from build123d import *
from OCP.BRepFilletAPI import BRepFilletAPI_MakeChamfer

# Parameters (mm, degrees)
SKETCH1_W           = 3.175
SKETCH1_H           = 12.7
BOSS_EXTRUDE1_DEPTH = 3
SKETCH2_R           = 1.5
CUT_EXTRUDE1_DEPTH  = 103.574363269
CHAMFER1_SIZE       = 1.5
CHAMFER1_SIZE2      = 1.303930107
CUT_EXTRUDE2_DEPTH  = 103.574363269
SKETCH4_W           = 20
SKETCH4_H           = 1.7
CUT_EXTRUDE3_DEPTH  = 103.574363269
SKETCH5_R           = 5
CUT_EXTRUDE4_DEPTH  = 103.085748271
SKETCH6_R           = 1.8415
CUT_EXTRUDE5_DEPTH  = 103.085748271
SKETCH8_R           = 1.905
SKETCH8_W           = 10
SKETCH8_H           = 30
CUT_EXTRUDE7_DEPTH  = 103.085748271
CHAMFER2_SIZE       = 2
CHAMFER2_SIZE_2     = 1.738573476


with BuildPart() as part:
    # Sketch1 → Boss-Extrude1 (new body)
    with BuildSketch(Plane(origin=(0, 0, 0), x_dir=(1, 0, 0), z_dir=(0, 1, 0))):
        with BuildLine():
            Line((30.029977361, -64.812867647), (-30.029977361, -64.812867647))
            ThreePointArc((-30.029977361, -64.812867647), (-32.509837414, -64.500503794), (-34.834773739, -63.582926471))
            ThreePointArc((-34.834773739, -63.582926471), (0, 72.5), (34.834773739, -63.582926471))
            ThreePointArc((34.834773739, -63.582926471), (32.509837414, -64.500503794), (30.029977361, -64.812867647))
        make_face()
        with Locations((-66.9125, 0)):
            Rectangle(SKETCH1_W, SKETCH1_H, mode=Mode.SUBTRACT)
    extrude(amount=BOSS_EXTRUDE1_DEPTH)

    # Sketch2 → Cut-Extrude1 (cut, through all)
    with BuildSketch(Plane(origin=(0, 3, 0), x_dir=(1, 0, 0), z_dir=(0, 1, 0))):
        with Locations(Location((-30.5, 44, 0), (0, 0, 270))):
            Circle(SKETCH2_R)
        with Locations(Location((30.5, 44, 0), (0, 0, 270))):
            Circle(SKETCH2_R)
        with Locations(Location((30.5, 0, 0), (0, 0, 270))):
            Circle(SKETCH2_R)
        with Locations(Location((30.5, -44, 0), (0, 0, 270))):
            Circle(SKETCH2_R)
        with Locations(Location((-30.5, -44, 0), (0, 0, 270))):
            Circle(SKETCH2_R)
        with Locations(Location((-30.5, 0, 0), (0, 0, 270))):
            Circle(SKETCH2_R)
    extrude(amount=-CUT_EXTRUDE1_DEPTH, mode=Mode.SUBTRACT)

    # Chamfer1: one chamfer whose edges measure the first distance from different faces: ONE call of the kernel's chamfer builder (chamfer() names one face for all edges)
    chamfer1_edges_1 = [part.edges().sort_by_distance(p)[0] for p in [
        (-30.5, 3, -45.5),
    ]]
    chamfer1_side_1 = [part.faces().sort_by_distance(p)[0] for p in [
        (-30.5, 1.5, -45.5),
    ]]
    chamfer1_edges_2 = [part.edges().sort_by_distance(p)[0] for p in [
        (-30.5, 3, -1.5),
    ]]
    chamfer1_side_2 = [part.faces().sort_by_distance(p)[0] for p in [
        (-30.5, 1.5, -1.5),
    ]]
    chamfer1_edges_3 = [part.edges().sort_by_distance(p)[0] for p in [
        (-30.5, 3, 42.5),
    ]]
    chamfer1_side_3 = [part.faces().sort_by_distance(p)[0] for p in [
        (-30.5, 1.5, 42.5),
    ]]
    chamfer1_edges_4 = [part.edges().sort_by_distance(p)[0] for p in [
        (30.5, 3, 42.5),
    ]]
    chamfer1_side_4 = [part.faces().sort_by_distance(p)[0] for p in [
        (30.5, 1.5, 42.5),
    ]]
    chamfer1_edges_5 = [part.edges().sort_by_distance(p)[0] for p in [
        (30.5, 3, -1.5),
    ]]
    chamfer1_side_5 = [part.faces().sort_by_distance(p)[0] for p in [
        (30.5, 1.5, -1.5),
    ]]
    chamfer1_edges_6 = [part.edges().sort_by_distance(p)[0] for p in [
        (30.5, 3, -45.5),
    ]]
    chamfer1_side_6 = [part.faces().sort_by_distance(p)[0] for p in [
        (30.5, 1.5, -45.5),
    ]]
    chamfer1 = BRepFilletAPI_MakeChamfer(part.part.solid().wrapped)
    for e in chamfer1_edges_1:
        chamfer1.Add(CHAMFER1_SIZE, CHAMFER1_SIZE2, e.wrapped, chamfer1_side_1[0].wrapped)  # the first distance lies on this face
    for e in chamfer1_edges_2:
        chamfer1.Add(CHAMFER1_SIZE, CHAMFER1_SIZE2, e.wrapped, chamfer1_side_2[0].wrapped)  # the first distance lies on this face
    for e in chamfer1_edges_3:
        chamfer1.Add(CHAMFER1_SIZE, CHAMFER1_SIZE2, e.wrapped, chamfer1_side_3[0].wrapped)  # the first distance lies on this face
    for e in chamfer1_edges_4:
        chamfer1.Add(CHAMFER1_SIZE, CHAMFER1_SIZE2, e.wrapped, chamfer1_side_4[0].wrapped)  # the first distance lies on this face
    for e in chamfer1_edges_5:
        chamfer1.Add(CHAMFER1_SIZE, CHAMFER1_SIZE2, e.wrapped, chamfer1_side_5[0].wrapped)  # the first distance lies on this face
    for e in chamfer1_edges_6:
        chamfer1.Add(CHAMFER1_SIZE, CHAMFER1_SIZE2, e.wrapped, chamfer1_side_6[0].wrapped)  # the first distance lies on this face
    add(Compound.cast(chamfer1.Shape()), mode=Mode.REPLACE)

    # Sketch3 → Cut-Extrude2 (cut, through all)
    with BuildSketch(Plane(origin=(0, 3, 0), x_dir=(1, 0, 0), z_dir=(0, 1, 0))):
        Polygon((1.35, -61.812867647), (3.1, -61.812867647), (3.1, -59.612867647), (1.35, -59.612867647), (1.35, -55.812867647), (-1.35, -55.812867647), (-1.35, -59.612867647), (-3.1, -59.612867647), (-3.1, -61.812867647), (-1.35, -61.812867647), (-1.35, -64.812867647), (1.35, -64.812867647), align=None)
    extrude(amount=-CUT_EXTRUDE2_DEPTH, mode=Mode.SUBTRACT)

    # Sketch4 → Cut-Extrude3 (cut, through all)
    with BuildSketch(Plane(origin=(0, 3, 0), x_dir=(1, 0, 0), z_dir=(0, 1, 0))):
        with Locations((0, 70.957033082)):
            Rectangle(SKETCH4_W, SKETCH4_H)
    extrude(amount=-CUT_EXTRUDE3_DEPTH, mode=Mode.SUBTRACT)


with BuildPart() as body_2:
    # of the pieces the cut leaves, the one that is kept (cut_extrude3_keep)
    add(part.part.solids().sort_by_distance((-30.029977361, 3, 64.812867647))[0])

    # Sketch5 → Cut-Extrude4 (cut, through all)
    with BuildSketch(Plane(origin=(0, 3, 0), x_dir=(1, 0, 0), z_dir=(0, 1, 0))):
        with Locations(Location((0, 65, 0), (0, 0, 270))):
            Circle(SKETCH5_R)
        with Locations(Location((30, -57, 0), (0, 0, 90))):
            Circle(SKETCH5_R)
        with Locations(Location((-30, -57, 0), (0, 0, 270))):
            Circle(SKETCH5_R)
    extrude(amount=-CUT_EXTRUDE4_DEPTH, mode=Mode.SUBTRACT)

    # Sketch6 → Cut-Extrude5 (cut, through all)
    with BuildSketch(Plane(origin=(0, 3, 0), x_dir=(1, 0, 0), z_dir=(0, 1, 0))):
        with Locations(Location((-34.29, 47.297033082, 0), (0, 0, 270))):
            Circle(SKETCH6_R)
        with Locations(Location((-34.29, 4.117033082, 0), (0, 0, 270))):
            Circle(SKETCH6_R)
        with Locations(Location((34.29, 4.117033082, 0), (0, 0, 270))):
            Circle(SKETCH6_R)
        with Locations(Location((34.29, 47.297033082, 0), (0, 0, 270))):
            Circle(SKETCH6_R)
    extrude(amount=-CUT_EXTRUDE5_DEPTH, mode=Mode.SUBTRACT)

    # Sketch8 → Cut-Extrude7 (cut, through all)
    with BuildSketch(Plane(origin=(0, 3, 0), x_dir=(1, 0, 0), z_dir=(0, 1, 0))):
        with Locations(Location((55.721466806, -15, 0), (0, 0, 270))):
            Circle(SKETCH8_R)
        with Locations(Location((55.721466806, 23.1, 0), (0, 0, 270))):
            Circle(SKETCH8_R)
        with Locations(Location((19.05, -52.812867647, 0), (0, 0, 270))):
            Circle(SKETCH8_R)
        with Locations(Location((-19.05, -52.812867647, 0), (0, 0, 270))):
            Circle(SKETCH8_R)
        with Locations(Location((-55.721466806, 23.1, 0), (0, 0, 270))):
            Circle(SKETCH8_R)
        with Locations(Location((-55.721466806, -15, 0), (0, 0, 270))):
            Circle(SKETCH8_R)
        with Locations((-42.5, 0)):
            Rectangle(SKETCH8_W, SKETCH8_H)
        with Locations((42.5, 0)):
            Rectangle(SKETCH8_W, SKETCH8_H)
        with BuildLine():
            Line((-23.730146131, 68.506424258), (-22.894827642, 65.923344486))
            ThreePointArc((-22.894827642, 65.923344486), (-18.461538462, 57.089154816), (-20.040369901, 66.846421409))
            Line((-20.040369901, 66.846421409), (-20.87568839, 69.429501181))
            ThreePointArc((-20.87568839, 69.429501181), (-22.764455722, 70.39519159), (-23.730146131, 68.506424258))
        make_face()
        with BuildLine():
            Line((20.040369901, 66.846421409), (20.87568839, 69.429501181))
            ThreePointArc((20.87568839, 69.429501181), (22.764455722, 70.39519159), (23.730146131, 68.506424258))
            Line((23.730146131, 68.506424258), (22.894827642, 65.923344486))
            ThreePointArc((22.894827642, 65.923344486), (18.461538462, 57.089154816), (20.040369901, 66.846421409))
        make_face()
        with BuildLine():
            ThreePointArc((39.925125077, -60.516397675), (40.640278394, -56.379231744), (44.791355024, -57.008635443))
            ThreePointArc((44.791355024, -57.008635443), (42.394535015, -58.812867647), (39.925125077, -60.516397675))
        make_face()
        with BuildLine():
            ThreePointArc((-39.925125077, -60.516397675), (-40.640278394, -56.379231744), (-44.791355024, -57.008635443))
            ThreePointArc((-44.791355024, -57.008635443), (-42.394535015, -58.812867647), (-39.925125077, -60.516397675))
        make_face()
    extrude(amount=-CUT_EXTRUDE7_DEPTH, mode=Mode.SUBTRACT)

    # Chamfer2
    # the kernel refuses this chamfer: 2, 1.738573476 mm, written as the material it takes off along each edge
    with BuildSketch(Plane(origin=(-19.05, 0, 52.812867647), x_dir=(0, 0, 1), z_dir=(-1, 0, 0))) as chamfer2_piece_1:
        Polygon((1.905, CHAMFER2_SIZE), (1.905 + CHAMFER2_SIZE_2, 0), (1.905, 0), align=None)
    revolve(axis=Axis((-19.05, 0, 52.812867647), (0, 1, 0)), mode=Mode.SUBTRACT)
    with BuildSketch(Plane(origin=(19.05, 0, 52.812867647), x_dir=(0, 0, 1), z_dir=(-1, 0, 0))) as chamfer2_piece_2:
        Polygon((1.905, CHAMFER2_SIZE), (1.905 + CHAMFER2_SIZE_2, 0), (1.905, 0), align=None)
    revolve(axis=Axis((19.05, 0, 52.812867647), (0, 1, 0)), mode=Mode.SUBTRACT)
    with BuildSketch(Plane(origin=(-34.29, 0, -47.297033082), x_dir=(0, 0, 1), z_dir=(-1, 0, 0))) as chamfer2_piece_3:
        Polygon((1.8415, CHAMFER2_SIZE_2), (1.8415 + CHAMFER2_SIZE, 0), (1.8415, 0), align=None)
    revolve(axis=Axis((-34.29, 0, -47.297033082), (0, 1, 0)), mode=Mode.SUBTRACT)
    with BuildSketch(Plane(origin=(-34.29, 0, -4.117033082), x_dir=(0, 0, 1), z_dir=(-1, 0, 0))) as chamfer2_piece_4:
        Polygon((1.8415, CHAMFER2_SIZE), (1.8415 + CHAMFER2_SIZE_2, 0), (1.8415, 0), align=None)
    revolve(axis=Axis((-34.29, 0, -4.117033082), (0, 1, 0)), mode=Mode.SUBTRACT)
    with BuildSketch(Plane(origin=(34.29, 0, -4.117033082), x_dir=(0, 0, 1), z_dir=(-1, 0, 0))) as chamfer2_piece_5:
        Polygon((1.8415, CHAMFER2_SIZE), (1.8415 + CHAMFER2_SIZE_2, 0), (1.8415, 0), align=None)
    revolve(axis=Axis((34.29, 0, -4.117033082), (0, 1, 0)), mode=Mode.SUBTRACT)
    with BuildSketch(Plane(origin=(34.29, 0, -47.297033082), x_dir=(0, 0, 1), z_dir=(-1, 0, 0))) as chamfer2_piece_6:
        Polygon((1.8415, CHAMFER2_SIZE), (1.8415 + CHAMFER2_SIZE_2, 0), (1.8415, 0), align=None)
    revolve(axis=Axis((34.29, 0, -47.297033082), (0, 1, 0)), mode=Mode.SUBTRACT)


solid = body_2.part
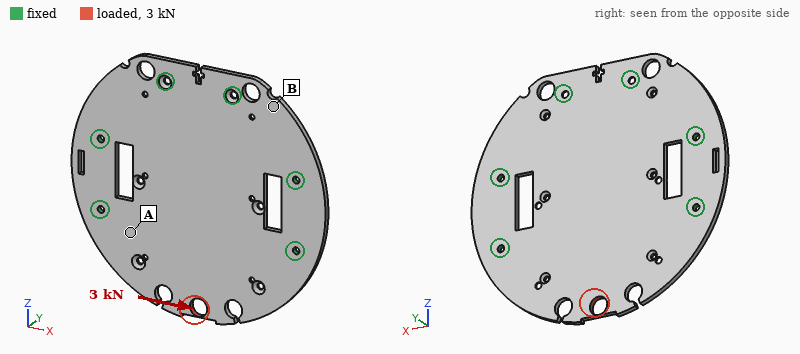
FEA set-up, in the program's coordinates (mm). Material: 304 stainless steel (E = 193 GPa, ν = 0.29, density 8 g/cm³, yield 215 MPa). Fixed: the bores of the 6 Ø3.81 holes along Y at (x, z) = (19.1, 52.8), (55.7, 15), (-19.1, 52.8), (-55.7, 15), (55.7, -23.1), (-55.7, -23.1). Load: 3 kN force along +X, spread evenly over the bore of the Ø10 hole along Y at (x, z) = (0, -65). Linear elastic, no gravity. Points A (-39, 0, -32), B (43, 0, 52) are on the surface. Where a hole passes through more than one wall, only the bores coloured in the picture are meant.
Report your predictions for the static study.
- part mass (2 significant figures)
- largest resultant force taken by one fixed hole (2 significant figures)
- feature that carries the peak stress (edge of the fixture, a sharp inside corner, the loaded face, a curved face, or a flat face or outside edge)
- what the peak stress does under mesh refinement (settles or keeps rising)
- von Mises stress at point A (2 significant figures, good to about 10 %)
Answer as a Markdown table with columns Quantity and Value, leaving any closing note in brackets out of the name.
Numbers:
| Quantity | Value |
|---|---|
| part mass | 360 g |
| largest resultant force taken by one fixed hole | 1.6 kN |
| feature that carries the peak stress | a sharp inside corner |
| what the peak stress does under mesh refinement | keeps rising |
| von Mises stress at point A | 24 MPa |
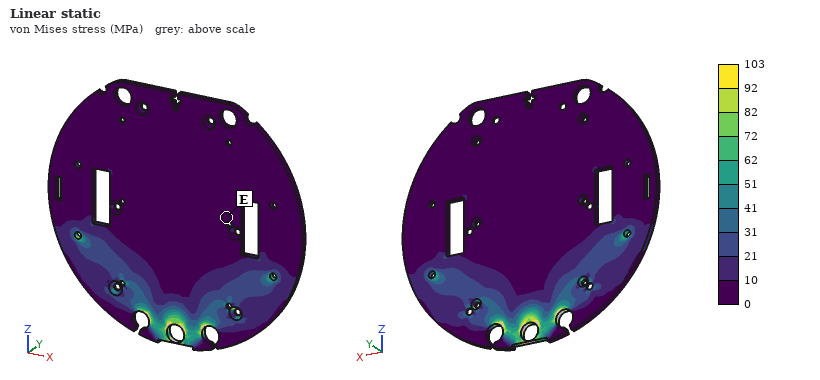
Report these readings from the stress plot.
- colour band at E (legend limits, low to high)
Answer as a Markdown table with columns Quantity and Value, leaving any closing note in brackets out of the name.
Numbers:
| Quantity | Value |
|---|---|
| colour band at E | 0 to 10 MPa |
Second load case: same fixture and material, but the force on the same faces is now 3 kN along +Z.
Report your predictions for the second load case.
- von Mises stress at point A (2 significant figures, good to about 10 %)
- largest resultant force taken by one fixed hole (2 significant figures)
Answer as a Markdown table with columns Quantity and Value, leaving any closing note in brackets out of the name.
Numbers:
| Quantity | Value |
|---|---|
| von Mises stress at point A | 12 MPa |
| largest resultant force taken by one fixed hole | 660 N |
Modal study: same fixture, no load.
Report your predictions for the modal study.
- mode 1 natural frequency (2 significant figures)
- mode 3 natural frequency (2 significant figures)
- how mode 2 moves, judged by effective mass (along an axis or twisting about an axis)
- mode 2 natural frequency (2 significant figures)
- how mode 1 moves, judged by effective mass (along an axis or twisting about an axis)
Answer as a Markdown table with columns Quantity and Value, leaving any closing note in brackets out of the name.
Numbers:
| Quantity | Value |
|---|---|
| mode 1 natural frequency | 770 Hz |
| mode 3 natural frequency | 1900 Hz |
| how mode 2 moves, judged by effective mass | along Y |
| mode 2 natural frequency | 1500 Hz |
| how mode 1 moves, judged by effective mass | along Y |
